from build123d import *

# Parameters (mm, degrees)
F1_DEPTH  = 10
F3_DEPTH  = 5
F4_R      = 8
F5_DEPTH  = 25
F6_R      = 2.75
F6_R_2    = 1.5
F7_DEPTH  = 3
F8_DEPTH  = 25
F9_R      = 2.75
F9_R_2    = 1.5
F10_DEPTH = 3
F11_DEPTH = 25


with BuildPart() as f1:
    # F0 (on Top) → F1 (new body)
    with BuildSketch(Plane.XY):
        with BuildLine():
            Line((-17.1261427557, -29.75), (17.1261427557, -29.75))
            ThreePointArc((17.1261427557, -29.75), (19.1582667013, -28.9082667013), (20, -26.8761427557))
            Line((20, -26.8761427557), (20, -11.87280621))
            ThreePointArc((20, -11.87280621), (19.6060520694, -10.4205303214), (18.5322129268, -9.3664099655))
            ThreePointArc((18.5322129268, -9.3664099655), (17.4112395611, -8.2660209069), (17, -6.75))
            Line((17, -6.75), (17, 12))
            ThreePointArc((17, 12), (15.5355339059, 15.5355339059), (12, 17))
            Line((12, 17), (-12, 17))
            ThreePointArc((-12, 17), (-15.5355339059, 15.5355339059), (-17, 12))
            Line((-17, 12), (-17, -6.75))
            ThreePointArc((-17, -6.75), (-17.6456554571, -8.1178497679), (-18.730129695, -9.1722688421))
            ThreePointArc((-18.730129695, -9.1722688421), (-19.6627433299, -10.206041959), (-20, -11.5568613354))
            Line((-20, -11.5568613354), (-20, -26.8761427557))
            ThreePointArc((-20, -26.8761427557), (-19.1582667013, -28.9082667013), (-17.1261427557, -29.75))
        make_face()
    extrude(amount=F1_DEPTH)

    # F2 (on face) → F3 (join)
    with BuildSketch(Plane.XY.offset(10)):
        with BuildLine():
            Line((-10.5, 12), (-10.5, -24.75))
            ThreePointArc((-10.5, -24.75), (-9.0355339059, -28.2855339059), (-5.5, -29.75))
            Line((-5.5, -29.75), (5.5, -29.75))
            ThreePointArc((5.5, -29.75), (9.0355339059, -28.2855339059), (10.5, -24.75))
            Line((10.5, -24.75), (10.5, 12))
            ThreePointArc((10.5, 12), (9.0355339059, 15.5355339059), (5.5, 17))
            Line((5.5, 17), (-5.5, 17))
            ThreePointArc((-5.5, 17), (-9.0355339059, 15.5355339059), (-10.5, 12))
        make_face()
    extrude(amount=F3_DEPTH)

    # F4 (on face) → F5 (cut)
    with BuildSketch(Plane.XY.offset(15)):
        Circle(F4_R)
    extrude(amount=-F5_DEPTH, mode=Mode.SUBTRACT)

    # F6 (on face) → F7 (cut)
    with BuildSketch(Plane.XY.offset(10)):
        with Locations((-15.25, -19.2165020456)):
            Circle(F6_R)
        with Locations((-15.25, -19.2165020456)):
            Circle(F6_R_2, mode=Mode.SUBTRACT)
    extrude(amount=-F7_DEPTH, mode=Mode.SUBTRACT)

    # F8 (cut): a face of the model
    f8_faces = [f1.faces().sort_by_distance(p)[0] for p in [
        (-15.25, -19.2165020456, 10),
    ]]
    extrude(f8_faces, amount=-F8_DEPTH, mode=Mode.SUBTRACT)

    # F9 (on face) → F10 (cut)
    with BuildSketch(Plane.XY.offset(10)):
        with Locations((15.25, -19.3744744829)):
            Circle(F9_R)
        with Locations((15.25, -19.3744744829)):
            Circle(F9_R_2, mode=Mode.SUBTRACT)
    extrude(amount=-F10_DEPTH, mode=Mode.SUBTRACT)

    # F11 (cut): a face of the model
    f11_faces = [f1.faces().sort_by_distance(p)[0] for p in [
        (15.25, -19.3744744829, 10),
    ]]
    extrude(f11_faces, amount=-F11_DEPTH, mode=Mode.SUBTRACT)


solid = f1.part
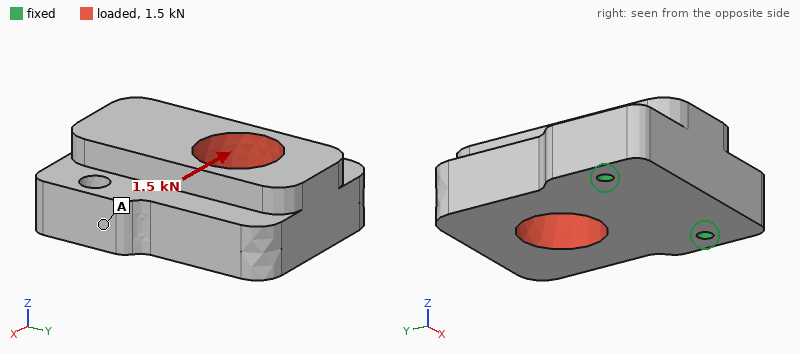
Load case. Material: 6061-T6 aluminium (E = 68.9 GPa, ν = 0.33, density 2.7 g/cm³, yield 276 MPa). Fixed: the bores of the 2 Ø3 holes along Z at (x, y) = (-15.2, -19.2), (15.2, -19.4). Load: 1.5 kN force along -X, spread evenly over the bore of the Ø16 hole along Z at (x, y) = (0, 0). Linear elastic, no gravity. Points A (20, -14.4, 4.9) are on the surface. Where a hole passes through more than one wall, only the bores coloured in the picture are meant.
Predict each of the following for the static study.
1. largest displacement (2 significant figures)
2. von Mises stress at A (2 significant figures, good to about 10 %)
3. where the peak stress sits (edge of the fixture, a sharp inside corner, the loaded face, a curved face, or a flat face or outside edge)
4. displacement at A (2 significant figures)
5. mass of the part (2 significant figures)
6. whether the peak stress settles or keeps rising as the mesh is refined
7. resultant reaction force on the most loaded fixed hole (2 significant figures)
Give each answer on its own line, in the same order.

11 µm
6.8 MPa
edge of the fixture
2.3 µm
50 g
keeps rising
1.2 kN
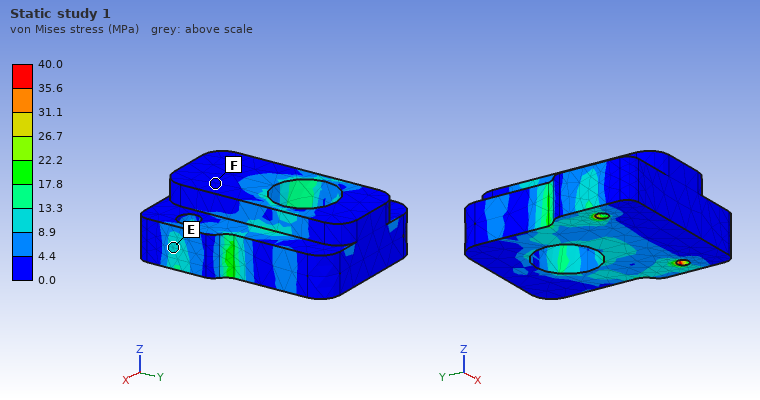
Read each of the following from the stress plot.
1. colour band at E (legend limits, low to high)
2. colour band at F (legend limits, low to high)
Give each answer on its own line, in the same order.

8.9 to 13.3 MPa
0.0 to 4.4 MPa
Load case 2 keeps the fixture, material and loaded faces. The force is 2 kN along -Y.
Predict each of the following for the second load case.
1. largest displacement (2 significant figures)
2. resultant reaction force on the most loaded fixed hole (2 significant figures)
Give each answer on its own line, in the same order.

25 µm
1.0 kN
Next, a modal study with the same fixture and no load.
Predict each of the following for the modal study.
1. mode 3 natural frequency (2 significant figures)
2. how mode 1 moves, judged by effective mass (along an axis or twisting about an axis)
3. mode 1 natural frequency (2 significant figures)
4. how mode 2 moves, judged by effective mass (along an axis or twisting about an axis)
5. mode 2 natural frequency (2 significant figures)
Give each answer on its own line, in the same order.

13 kHz
along Z
4100 Hz
along X
11 kHz
